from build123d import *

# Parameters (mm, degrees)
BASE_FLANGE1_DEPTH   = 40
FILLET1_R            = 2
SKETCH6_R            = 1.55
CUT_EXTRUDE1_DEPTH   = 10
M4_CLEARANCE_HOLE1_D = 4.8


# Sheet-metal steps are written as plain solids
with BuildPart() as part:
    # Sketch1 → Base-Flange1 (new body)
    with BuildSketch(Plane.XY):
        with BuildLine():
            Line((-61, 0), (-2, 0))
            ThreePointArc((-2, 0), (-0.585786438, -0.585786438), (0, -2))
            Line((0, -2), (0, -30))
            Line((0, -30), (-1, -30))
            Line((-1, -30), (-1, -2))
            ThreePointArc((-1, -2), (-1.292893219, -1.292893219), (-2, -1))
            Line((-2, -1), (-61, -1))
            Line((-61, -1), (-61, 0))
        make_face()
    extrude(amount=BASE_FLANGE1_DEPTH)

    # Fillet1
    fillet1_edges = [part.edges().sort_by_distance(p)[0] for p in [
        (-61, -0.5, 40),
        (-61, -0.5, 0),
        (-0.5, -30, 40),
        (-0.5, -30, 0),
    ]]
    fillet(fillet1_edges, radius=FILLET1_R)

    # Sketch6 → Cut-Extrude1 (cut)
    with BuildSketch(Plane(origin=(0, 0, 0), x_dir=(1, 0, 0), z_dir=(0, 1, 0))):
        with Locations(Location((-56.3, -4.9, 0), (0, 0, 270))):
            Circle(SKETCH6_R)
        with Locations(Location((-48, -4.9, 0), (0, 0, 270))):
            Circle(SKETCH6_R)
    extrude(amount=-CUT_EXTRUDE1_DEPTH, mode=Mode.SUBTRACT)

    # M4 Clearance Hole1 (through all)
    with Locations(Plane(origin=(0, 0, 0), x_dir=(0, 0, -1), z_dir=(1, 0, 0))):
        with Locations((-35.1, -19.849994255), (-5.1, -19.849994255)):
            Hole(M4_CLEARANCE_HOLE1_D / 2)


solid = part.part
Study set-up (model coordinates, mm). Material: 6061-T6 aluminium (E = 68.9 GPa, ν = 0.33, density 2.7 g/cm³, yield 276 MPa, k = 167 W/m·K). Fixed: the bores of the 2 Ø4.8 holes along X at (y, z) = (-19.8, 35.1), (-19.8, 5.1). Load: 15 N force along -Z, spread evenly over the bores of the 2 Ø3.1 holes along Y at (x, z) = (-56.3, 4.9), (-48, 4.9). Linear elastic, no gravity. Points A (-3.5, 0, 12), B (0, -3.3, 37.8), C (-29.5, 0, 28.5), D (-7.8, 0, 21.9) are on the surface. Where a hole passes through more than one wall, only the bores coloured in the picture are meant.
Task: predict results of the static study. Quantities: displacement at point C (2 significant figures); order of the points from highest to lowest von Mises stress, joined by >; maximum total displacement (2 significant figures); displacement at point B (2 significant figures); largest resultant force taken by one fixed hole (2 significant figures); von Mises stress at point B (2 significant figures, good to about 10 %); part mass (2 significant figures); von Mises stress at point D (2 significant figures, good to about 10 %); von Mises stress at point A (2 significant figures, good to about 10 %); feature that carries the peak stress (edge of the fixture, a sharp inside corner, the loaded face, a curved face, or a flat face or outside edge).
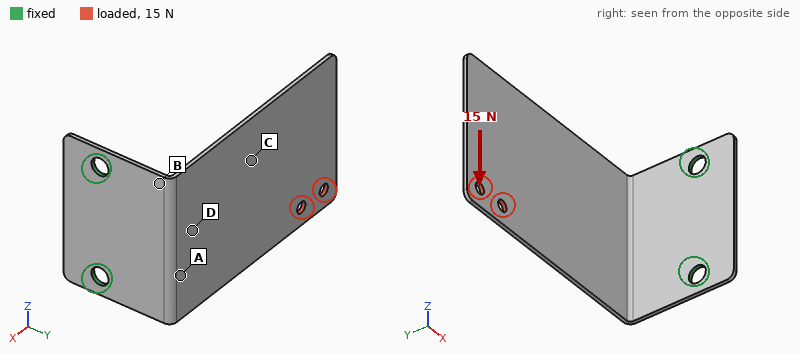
0.42 mm
B > A > D > C
0.89 mm
0.20 mm
28 N
47 MPa
9.5 g
18 MPa
32 MPa
a flat face or outside edge
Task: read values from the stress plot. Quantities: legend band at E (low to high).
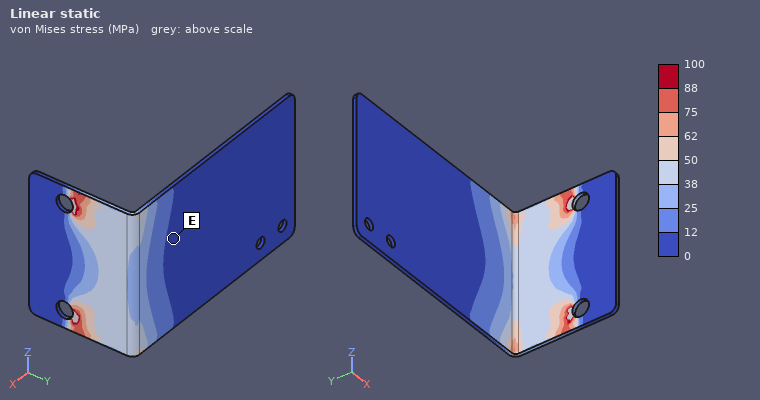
0 to 12 MPa
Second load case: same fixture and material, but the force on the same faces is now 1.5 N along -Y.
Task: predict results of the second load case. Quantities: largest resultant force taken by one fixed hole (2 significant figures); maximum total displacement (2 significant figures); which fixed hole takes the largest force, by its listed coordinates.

1.6 N
0.75 mm
(-19.8, 5.1)
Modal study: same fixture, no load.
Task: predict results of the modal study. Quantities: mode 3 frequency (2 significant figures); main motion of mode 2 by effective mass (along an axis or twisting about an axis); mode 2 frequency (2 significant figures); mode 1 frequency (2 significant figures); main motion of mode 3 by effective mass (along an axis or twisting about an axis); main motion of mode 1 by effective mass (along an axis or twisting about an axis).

750 Hz
along Z
400 Hz
160 Hz
twisting about X
along Y
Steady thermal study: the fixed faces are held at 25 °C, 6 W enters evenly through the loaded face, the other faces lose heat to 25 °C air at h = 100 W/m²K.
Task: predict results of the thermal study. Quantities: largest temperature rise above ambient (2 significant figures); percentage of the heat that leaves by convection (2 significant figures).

34 K
88 %
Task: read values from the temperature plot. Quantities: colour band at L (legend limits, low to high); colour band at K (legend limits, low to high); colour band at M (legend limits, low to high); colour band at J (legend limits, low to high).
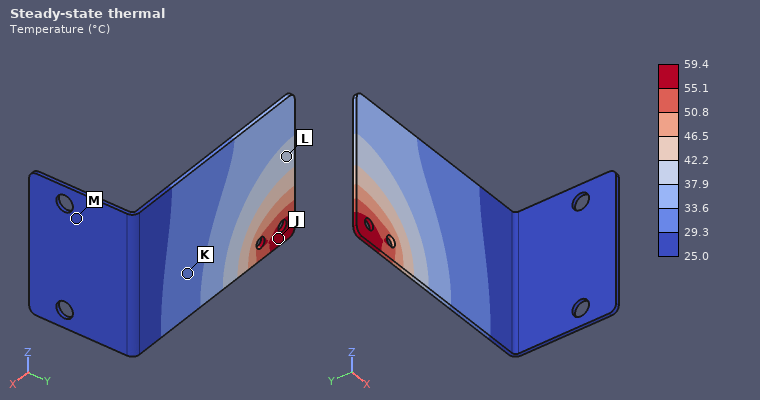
37.9 to 42.2 °C
29.3 to 33.6 °C
25.0 to 29.3 °C
55.1 to 59.4 °C
